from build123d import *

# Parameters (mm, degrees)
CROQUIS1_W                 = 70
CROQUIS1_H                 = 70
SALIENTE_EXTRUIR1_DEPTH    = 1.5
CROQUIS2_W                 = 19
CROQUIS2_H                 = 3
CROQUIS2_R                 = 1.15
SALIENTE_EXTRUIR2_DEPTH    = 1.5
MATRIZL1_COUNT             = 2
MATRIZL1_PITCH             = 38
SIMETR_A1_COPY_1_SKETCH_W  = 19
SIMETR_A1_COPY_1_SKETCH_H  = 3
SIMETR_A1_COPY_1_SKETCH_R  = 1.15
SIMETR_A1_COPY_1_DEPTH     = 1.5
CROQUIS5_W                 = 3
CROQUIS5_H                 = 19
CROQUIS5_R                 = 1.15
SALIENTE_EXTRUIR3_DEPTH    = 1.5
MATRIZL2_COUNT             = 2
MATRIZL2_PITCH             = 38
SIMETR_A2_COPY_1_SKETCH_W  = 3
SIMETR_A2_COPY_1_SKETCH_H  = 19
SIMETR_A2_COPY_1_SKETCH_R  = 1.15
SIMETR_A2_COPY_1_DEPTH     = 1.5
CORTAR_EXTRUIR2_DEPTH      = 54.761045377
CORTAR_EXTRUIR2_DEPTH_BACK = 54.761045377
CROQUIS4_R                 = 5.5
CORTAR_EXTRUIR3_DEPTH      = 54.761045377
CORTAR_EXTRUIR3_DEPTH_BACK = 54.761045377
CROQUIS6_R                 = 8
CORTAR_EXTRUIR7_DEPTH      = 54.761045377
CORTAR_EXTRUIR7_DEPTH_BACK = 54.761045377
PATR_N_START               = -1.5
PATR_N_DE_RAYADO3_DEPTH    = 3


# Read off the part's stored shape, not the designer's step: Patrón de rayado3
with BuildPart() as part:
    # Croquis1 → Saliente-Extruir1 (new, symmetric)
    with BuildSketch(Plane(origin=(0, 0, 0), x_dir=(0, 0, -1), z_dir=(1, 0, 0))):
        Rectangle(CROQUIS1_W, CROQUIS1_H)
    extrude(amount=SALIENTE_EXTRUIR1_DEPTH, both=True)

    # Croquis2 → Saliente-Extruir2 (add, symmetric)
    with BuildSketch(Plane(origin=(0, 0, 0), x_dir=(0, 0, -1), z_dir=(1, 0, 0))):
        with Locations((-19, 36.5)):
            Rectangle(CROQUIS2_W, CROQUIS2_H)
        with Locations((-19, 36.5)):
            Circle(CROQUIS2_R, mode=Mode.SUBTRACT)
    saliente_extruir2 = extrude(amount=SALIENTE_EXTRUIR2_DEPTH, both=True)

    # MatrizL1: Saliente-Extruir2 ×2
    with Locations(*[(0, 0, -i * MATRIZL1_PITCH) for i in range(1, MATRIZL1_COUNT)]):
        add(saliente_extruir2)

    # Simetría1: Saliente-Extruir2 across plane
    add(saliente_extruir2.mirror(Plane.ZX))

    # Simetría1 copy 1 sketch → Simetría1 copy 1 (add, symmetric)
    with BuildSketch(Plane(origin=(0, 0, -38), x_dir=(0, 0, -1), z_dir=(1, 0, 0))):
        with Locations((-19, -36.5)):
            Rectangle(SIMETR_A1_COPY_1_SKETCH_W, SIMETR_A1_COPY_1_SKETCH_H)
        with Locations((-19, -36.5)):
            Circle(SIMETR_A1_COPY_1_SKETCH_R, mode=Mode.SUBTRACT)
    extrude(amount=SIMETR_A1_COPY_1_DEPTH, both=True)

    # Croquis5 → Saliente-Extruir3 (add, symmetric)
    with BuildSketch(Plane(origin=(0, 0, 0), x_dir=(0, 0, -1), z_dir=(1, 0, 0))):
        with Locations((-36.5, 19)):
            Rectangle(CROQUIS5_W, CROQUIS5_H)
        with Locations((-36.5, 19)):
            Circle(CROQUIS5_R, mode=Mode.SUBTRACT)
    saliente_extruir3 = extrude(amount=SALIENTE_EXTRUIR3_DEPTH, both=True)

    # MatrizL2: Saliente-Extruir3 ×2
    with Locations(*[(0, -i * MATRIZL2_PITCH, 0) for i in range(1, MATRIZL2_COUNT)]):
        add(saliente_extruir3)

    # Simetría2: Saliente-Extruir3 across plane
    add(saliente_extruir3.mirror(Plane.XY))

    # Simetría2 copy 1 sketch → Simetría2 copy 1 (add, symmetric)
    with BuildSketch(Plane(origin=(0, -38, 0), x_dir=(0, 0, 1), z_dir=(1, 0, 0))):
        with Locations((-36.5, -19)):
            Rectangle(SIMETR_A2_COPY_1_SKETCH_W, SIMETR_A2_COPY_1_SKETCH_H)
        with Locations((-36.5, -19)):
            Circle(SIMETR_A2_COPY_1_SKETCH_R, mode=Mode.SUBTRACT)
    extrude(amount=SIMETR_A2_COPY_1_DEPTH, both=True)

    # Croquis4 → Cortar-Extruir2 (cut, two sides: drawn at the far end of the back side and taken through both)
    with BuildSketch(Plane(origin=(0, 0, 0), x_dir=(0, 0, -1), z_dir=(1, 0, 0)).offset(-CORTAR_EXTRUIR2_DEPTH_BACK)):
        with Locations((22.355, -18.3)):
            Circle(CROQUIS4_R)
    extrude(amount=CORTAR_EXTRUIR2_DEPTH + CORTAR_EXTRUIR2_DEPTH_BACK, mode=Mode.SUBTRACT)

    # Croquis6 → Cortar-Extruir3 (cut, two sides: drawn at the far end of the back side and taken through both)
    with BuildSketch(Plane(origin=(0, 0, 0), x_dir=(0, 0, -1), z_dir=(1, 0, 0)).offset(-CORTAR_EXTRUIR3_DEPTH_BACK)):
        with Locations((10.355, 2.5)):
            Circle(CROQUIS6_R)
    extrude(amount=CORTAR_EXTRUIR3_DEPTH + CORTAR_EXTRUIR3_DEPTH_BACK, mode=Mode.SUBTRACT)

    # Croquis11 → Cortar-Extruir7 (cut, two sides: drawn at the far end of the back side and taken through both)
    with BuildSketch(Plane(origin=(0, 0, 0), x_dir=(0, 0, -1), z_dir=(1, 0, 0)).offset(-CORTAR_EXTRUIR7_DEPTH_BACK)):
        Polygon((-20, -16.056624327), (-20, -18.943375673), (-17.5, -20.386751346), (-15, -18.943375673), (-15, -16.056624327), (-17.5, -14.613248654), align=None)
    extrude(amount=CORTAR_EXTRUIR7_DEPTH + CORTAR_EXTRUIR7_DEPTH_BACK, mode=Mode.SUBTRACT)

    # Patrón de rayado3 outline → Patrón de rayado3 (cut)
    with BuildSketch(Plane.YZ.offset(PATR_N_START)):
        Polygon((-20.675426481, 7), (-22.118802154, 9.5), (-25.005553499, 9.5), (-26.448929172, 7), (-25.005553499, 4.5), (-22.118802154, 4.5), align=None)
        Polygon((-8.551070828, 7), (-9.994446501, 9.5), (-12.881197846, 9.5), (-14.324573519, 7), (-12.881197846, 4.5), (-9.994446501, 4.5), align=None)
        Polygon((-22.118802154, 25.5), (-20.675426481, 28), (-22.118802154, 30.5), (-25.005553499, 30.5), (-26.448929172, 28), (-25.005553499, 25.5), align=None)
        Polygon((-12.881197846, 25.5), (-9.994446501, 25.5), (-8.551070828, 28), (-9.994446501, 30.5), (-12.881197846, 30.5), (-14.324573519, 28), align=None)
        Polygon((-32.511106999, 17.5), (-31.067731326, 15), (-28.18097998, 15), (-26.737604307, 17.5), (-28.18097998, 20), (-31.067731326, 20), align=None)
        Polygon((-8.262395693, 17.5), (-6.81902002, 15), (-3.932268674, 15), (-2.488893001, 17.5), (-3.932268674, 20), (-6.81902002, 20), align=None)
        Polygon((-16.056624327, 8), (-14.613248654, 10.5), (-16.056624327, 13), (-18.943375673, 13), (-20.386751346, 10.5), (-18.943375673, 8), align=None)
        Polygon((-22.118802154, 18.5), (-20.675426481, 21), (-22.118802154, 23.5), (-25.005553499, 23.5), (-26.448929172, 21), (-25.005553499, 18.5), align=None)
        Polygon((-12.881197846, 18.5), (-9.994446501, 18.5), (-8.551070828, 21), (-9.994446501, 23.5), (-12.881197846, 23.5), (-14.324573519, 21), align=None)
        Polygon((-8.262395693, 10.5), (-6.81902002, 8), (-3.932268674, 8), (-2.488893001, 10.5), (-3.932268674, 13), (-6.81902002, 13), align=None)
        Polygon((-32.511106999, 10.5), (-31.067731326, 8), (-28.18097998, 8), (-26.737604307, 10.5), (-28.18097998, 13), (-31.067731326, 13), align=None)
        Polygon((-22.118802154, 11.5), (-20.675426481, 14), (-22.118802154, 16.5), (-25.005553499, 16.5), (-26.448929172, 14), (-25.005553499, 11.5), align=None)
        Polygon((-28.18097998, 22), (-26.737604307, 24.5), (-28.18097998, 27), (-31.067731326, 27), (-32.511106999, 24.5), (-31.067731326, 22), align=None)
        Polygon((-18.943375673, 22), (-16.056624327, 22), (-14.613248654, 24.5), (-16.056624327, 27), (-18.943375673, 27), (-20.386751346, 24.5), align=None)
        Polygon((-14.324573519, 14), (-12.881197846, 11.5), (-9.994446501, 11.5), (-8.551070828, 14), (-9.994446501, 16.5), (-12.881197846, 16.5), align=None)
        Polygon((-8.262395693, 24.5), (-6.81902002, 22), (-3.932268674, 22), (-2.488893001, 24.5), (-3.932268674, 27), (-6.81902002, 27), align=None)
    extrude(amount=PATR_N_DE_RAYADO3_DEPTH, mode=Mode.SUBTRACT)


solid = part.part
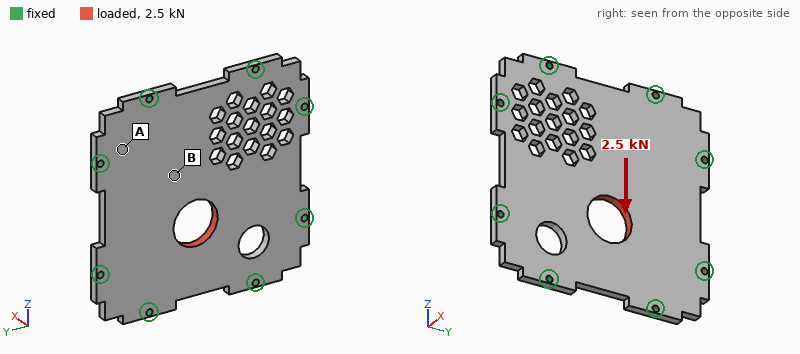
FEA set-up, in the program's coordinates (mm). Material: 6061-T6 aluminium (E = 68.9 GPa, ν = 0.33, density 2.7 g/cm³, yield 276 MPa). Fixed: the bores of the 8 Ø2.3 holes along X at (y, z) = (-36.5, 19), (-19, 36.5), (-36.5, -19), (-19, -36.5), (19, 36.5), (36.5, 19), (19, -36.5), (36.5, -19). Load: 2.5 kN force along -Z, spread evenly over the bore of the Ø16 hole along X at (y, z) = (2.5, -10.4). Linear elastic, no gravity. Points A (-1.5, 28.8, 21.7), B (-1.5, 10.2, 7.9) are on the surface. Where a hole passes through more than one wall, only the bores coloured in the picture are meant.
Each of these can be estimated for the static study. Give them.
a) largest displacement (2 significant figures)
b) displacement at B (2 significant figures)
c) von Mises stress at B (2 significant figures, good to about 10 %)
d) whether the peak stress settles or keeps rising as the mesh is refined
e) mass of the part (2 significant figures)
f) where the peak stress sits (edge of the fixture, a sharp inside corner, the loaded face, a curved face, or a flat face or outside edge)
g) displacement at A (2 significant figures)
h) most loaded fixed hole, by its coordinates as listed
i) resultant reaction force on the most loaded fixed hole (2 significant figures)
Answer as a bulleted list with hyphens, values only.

- 10 µm
- 5.2 µm
- 11 MPa
- keeps rising
- 38 g
- edge of the fixture
- 1.7 µm
- (19, -36.5)
- 740 N
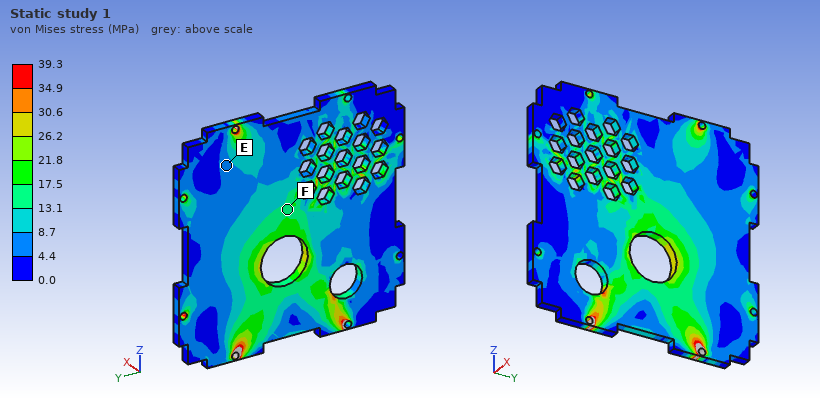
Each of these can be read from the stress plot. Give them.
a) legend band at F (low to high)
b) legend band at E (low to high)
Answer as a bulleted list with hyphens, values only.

- 13.1 to 17.5 MPa
- 4.4 to 8.7 MPa
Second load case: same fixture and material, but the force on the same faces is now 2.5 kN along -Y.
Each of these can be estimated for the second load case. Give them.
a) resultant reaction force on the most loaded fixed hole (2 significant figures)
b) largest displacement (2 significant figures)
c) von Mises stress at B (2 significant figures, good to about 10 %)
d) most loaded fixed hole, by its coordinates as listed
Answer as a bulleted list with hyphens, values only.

- 650 N
- 9.1 µm
- 7.5 MPa
- (36.5, -19)
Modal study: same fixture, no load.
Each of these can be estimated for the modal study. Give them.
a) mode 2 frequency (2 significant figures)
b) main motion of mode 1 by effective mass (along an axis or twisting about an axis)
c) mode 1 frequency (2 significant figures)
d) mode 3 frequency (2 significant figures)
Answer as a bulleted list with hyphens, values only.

- 6800 Hz
- along X
- 3300 Hz
- 6900 Hz
